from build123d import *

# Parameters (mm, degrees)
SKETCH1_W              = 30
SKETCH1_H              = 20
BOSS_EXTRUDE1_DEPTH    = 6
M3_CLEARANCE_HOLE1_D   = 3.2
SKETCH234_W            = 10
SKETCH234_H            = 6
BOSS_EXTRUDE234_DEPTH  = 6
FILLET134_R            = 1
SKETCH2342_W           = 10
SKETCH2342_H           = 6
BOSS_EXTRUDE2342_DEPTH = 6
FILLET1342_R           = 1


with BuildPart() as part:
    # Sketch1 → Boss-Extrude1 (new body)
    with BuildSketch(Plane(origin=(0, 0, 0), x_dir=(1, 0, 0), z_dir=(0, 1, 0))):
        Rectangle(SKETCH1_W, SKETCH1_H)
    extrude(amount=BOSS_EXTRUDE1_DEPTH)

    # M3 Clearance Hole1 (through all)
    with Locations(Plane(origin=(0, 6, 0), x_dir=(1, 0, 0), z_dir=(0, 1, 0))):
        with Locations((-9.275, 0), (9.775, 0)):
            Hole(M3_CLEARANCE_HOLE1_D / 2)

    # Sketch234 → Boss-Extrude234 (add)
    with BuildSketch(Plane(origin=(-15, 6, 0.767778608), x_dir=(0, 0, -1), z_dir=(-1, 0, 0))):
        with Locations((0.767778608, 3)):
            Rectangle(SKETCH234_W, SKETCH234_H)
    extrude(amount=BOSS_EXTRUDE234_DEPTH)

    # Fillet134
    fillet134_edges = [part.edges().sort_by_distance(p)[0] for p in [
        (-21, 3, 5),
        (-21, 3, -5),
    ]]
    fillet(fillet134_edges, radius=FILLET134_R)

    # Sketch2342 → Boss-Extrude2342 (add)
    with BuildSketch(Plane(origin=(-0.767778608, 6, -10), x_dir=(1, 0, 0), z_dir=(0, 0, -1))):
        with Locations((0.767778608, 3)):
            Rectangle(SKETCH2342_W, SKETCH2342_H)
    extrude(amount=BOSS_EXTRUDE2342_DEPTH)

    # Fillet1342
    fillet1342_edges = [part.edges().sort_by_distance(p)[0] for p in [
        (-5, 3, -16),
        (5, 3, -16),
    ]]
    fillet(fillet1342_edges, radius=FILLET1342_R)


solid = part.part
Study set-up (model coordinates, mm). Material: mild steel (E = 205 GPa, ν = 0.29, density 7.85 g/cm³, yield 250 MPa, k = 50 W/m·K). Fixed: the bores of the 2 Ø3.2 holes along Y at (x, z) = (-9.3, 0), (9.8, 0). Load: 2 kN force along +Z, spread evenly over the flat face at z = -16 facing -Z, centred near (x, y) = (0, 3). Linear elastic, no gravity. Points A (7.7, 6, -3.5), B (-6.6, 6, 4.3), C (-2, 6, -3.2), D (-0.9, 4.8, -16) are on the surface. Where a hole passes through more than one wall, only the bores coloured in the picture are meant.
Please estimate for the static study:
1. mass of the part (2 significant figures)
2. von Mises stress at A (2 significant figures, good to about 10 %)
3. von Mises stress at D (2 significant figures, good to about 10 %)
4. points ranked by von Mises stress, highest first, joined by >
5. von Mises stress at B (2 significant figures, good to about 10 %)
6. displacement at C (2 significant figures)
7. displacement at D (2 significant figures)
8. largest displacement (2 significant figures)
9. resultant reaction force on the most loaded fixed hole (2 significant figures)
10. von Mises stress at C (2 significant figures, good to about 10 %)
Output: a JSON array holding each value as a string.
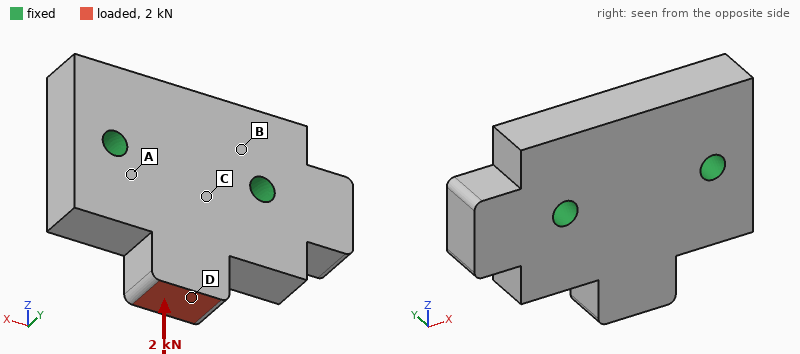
["33 g", "25 MPa", "36 MPa", "D > A > C > B", "11 MPa", "0.95 µm", "2.7 µm", "2.7 µm", "1.1 kN", "16 MPa"]
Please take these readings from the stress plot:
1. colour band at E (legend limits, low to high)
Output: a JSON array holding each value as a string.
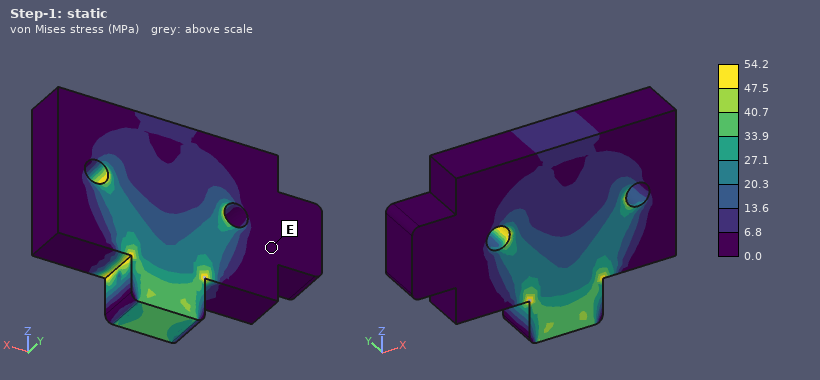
["0.0 to 6.8 MPa"]
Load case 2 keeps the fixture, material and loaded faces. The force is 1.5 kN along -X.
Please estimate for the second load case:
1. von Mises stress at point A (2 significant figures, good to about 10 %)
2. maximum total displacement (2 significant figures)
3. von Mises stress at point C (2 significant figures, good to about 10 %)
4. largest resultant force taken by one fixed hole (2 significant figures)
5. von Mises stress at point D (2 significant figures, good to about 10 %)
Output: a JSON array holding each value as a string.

["39 MPa", "7.7 µm", "10 MPa", "1.4 kN", "55 MPa"]
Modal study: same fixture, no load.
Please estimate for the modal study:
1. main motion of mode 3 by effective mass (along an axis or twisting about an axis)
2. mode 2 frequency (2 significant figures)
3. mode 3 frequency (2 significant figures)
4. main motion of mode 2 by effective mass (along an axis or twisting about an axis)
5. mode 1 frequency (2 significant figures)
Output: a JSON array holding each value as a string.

["along Y", "33 kHz", "36 kHz", "twisting about Z", "21 kHz"]
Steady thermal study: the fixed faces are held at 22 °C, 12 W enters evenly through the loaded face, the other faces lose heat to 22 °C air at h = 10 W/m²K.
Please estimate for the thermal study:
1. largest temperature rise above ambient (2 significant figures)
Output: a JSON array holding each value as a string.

["51 K"]
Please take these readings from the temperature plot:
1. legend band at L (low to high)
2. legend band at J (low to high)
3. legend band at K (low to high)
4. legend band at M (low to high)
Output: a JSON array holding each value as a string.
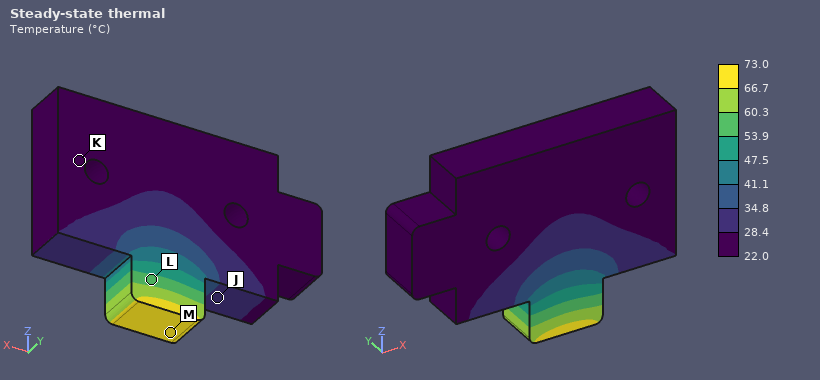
["53.9 to 60.3 °C", "28.4 to 34.8 °C", "22.0 to 28.4 °C", "66.7 to 73.0 °C"]
